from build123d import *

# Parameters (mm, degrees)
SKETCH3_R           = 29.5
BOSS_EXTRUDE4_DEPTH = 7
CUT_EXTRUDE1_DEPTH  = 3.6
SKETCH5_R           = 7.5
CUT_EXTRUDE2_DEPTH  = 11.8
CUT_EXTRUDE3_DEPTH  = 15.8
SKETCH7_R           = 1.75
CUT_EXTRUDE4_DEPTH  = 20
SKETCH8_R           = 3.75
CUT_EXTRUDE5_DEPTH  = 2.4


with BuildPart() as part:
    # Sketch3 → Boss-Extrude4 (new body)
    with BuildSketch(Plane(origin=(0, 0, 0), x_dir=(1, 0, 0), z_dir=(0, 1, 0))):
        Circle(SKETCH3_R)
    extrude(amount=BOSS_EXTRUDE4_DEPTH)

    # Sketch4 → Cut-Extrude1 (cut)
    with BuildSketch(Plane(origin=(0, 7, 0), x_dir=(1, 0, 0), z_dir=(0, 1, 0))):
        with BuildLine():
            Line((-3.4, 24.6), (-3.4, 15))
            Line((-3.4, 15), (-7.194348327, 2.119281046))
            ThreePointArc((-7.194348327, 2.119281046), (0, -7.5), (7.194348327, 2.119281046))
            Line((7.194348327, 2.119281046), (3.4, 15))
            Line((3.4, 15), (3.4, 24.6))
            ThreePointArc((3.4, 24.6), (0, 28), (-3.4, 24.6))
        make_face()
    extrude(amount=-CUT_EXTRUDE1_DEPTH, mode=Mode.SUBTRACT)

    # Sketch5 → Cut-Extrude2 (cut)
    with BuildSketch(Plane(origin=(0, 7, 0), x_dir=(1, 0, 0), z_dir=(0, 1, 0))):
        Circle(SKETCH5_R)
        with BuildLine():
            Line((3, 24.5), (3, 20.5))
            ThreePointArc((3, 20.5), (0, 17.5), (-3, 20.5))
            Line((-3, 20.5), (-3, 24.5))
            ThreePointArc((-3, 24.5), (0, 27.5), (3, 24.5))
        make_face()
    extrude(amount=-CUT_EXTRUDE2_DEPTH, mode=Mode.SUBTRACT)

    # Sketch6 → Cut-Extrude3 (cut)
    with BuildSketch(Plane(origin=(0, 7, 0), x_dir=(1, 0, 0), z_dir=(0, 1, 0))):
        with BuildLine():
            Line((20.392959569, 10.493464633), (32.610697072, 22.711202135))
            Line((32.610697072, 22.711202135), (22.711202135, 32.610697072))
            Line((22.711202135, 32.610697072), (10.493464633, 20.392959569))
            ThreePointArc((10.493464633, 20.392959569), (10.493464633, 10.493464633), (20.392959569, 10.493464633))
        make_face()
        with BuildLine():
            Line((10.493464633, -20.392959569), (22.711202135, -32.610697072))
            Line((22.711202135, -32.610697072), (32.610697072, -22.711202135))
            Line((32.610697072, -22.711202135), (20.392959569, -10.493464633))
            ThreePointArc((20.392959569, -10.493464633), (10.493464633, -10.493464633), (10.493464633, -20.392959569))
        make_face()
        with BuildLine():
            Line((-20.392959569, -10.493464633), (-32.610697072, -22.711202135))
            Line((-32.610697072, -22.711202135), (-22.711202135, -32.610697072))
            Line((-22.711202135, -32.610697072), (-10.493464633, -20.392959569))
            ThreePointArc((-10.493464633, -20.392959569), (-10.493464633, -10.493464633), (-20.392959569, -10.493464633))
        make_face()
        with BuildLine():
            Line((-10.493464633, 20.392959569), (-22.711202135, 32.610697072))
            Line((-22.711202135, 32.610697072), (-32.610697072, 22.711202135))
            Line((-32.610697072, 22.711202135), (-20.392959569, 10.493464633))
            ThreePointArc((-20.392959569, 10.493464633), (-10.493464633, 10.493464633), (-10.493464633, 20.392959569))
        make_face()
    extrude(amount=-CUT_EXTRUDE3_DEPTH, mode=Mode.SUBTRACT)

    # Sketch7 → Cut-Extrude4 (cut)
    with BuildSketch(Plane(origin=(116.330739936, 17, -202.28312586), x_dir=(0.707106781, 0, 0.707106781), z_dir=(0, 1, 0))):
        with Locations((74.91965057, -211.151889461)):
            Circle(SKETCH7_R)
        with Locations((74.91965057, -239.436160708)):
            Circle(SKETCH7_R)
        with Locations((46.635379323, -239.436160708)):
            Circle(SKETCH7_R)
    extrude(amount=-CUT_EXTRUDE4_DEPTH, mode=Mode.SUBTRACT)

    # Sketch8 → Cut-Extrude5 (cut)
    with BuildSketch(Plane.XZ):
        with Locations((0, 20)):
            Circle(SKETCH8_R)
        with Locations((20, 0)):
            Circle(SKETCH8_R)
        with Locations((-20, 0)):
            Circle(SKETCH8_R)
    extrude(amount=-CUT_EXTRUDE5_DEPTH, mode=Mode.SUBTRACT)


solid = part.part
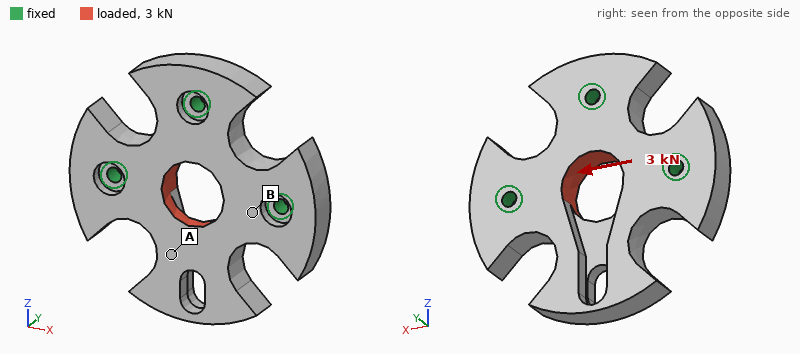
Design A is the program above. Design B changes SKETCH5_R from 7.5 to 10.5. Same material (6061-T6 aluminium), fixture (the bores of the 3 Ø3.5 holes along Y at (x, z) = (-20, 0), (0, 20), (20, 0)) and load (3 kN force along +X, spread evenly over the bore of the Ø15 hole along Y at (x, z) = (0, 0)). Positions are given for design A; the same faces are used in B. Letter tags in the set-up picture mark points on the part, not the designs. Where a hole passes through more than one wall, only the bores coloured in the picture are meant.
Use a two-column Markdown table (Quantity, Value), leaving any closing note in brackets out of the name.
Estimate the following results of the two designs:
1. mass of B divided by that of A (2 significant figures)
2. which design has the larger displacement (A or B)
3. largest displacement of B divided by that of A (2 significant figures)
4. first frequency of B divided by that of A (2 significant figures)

| Quantity | Value |
|---|---|
| mass of B divided by that of A | 0.91 |
| which design has the larger displacement | B |
| largest displacement of B divided by that of A | 1.1 |
| first frequency of B divided by that of A | 0.87 |
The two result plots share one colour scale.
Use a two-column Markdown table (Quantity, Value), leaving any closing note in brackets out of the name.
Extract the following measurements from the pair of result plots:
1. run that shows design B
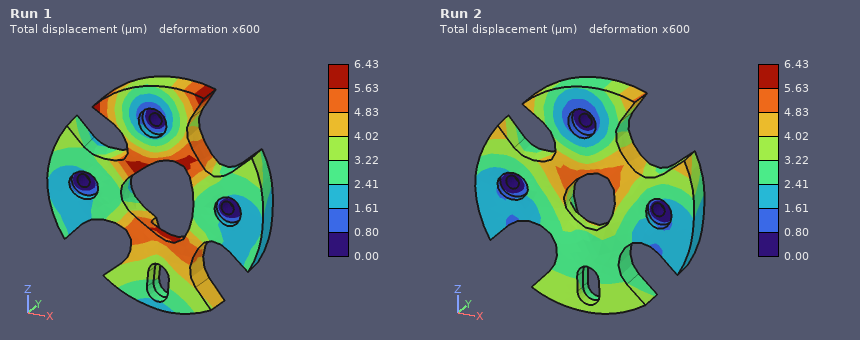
| Quantity | Value |
|---|---|
| run that shows design B | Run 1 |
